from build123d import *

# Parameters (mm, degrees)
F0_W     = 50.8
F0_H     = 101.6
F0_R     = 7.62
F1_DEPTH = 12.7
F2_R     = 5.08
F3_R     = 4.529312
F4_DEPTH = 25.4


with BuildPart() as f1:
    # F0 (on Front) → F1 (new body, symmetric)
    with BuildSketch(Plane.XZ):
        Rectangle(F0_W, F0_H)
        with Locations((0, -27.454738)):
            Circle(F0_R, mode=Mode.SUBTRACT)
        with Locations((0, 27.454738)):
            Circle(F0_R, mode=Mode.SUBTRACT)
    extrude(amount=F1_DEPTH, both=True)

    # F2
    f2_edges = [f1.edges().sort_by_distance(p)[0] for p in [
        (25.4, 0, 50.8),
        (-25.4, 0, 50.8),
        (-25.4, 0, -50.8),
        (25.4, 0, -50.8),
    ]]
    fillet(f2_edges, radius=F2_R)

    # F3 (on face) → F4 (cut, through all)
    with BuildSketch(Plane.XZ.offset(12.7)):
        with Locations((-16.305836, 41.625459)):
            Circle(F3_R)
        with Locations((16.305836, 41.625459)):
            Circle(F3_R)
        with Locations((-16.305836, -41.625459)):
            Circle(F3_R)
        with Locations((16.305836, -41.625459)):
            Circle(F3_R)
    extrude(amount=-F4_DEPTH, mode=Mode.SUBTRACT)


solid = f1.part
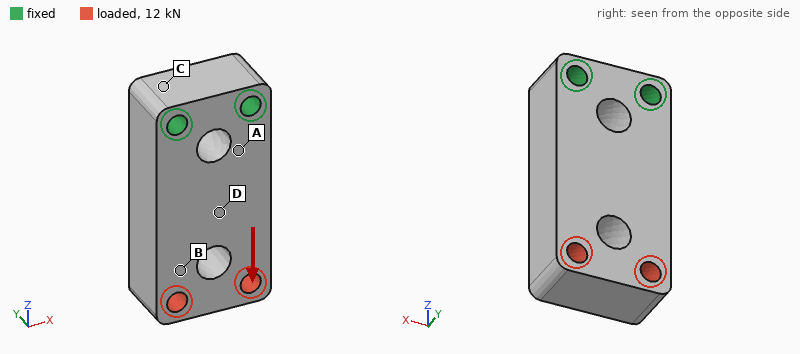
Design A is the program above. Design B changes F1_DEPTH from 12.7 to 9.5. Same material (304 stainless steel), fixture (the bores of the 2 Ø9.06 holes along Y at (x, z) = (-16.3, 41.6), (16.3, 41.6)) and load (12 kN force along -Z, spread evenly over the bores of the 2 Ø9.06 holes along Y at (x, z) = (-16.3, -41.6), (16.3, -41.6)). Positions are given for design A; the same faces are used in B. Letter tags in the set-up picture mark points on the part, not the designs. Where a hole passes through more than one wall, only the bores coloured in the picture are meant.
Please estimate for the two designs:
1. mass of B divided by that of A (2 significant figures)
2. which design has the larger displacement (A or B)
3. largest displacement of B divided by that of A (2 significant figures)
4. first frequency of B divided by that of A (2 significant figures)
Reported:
0.75
B
1.3
0.77
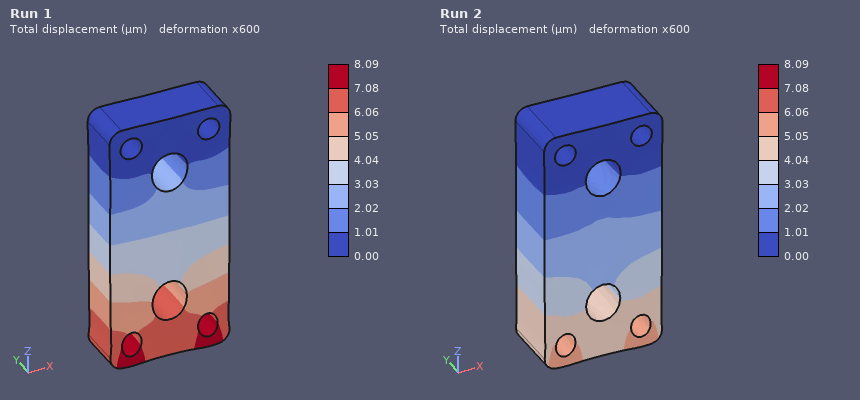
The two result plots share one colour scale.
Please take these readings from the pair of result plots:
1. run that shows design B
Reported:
Run 1
